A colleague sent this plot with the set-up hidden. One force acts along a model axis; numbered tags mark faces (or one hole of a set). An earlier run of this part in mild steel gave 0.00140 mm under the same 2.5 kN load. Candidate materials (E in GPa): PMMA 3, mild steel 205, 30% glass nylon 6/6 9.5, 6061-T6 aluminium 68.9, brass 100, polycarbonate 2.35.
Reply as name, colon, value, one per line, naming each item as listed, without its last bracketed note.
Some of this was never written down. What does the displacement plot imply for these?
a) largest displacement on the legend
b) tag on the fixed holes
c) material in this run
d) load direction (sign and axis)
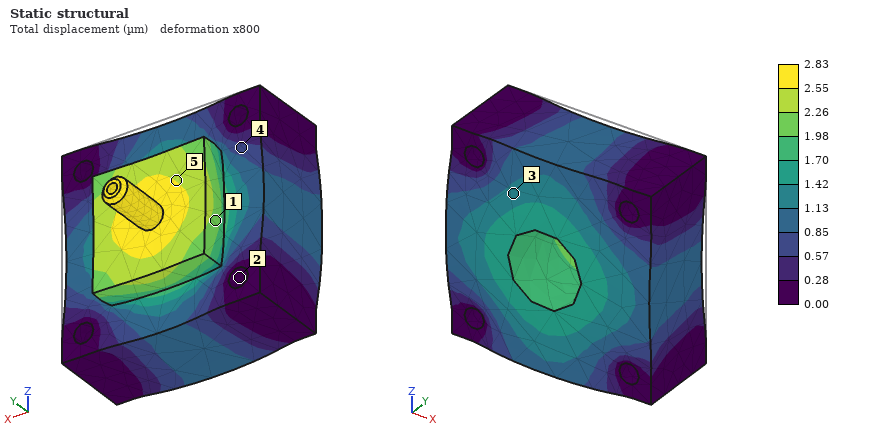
largest displacement on the legend: 2.83 µm
tag on the fixed holes: 2
material in this run: brass
load direction: -Y
